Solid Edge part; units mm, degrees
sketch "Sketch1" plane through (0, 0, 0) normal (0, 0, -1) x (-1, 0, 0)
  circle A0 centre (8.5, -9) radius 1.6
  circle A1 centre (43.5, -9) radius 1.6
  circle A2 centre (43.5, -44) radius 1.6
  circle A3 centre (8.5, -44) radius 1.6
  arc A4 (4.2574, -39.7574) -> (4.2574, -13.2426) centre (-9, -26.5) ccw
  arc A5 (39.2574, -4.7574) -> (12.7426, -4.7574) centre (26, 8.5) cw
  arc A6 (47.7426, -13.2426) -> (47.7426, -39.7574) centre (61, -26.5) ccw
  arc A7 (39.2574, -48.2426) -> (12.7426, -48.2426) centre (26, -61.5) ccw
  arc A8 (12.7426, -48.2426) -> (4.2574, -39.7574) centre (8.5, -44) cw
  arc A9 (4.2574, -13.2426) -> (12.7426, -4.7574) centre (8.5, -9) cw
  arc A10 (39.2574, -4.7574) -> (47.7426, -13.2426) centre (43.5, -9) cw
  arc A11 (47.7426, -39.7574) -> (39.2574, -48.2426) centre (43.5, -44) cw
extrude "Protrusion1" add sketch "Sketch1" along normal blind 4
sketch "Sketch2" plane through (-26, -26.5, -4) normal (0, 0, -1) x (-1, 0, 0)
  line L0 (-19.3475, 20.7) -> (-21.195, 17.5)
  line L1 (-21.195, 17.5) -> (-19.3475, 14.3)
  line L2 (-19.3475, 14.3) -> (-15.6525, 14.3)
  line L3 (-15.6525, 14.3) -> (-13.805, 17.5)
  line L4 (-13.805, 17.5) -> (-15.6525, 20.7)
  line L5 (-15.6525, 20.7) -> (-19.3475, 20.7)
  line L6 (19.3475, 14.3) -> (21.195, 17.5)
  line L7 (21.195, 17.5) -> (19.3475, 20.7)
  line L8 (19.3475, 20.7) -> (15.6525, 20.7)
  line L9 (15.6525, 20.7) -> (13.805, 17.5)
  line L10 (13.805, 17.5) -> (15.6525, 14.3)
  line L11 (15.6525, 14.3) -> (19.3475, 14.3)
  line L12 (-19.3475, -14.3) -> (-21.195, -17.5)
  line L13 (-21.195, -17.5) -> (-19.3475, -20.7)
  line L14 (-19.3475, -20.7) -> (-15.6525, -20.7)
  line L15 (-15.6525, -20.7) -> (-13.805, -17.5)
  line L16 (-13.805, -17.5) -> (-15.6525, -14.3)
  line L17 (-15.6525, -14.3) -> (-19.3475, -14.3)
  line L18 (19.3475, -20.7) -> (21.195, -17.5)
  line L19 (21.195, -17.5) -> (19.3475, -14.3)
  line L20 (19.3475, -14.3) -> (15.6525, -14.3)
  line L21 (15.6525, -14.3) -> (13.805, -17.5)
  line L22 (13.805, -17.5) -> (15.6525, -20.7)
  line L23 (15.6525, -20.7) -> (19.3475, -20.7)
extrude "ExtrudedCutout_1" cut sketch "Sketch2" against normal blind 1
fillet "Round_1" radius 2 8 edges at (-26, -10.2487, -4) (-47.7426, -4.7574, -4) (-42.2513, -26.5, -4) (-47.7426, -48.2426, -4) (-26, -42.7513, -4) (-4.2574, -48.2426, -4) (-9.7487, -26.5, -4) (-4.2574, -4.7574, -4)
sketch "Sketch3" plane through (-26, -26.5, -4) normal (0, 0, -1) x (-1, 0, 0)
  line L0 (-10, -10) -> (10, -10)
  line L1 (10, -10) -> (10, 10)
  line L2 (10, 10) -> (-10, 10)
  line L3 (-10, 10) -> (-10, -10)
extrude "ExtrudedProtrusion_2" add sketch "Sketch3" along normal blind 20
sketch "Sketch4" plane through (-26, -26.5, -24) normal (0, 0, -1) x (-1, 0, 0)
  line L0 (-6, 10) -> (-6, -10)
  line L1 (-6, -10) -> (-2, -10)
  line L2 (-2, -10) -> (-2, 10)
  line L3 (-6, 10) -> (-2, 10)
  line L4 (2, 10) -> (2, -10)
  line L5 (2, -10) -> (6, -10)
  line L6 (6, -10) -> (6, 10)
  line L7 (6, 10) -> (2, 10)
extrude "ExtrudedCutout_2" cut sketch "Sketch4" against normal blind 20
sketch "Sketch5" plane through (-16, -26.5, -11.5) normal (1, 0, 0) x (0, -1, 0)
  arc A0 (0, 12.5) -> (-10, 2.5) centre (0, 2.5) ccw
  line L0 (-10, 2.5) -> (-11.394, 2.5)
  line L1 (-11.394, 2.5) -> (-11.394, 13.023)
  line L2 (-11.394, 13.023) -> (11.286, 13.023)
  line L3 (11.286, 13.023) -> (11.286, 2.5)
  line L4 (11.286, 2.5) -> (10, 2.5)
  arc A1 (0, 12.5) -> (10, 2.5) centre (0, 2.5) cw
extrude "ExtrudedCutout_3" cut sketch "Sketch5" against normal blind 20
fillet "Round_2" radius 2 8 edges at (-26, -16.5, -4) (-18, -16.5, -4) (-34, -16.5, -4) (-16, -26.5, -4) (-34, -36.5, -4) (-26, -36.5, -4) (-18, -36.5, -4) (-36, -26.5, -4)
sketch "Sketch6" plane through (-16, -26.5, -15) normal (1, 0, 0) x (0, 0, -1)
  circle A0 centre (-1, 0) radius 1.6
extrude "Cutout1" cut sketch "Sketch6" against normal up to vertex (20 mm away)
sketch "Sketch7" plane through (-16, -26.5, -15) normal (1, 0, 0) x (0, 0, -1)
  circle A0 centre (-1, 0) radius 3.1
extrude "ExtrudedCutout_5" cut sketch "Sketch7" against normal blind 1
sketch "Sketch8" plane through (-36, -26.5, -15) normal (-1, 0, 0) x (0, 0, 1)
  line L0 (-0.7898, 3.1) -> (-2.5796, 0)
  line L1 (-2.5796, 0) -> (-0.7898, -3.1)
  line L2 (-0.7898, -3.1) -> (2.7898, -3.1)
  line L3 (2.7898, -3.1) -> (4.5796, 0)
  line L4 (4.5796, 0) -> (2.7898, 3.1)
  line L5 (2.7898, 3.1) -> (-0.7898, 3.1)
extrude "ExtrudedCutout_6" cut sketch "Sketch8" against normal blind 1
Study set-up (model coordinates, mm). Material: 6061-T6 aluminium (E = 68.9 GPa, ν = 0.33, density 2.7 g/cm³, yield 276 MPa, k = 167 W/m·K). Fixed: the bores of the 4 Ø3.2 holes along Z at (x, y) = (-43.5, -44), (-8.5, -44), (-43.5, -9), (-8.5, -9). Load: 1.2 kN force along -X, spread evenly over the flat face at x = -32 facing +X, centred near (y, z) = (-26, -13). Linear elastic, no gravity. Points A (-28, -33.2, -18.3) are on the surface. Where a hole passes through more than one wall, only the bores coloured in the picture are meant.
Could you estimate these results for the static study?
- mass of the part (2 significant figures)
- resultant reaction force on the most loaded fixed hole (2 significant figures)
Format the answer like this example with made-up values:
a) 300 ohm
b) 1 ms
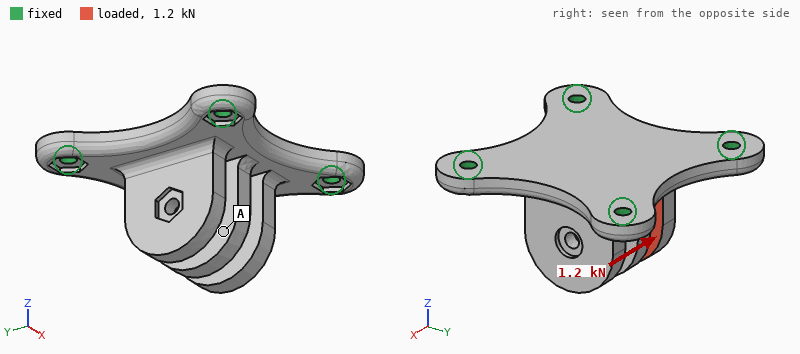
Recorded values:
a) 27 g
b) 460 N
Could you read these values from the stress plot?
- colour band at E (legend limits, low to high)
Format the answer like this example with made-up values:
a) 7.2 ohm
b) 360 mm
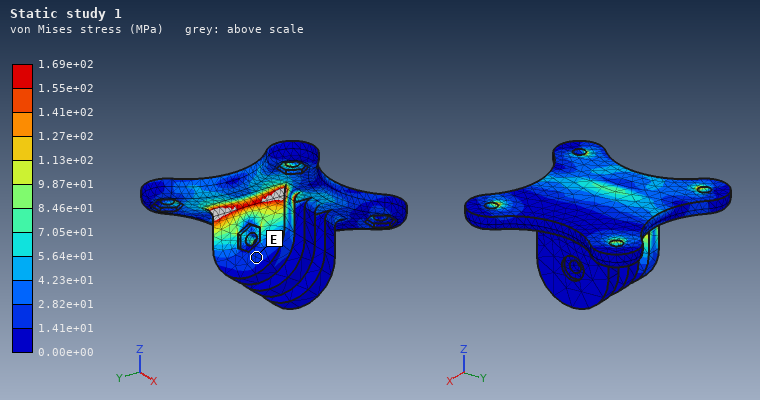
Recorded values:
a) 1.41e+01 to 2.82e+01 MPa
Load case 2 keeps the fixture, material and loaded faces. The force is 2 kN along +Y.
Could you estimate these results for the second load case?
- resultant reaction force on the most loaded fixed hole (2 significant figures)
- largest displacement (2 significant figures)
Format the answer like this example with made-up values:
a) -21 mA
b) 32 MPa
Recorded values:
a) 1.0 kN
b) 74 µm
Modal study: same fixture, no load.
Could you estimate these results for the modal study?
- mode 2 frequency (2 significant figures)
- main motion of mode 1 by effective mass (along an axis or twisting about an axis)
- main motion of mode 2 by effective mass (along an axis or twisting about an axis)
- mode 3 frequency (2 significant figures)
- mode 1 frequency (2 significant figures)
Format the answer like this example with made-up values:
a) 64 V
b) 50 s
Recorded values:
a) 7400 Hz
b) along Z
c) along X
d) 7900 Hz
e) 6100 Hz
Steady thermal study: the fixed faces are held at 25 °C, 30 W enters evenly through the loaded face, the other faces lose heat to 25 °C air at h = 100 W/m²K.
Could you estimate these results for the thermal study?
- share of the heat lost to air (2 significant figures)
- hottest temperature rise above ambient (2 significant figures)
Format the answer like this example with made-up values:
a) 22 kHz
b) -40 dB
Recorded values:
a) 18 %
b) 37 K
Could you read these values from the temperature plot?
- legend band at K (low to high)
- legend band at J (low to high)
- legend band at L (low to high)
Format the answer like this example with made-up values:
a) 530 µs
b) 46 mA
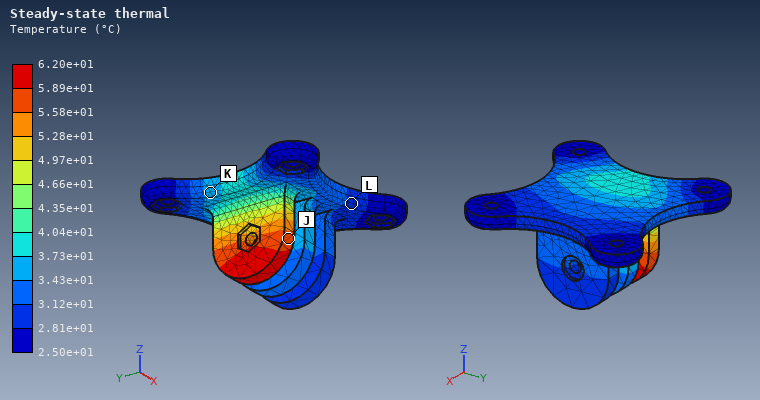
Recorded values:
a) 3.43e+01 to 3.73e+01 °C
b) 5.58e+01 to 5.89e+01 °C
c) 2.81e+01 to 3.12e+01 °C
